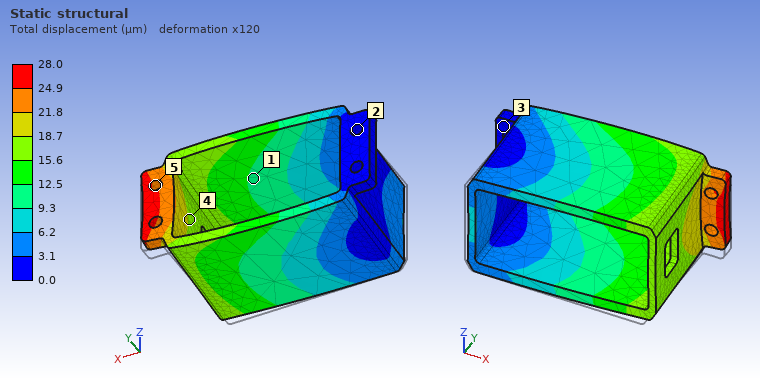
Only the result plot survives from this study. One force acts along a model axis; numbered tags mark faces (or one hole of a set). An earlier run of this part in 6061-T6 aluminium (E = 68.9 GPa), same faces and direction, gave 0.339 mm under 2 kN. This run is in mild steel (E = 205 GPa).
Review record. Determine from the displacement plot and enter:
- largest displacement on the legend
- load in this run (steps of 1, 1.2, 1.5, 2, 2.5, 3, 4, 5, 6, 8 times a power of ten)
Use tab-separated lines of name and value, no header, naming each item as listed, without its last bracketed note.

largest displacement on the legend	28.0 µm
load in this run	500 N
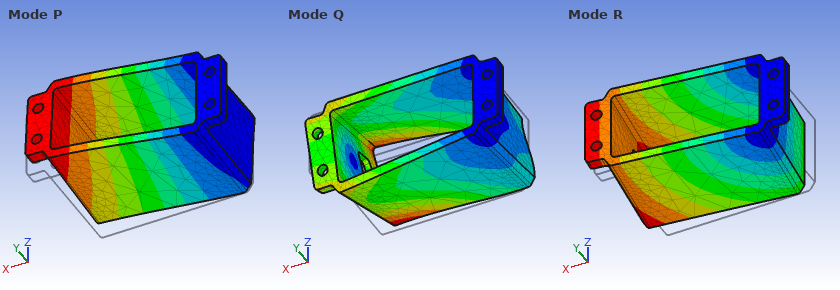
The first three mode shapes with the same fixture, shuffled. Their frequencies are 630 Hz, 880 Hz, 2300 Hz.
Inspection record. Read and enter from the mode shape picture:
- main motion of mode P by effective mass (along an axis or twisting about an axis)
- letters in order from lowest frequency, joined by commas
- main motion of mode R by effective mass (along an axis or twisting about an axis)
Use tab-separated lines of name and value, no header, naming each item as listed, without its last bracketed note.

main motion of mode P by effective mass	along Z
letters in order from lowest frequency, joined by commas	R, P, Q
main motion of mode R by effective mass	along Y
